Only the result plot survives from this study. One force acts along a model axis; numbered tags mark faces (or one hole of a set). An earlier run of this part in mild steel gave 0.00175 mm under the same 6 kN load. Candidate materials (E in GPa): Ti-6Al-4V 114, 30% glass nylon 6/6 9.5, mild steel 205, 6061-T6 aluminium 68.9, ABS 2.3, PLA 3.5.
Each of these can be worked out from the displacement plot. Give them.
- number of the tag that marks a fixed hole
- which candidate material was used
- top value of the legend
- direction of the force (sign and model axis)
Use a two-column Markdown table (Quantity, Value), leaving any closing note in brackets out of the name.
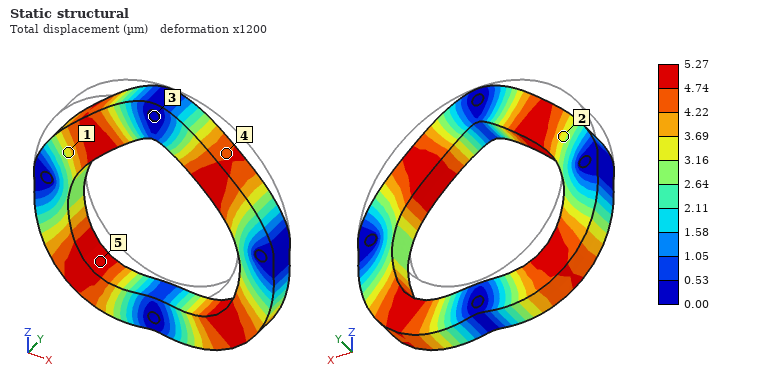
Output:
| Quantity | Value |
|---|---|
| number of the tag that marks a fixed hole | 3 |
| which candidate material was used | 6061-T6 aluminium |
| top value of the legend | 5.27 µm |
| direction of the force | -Z |
